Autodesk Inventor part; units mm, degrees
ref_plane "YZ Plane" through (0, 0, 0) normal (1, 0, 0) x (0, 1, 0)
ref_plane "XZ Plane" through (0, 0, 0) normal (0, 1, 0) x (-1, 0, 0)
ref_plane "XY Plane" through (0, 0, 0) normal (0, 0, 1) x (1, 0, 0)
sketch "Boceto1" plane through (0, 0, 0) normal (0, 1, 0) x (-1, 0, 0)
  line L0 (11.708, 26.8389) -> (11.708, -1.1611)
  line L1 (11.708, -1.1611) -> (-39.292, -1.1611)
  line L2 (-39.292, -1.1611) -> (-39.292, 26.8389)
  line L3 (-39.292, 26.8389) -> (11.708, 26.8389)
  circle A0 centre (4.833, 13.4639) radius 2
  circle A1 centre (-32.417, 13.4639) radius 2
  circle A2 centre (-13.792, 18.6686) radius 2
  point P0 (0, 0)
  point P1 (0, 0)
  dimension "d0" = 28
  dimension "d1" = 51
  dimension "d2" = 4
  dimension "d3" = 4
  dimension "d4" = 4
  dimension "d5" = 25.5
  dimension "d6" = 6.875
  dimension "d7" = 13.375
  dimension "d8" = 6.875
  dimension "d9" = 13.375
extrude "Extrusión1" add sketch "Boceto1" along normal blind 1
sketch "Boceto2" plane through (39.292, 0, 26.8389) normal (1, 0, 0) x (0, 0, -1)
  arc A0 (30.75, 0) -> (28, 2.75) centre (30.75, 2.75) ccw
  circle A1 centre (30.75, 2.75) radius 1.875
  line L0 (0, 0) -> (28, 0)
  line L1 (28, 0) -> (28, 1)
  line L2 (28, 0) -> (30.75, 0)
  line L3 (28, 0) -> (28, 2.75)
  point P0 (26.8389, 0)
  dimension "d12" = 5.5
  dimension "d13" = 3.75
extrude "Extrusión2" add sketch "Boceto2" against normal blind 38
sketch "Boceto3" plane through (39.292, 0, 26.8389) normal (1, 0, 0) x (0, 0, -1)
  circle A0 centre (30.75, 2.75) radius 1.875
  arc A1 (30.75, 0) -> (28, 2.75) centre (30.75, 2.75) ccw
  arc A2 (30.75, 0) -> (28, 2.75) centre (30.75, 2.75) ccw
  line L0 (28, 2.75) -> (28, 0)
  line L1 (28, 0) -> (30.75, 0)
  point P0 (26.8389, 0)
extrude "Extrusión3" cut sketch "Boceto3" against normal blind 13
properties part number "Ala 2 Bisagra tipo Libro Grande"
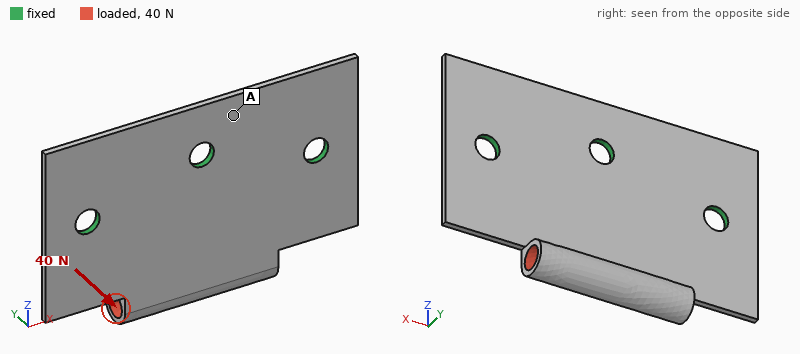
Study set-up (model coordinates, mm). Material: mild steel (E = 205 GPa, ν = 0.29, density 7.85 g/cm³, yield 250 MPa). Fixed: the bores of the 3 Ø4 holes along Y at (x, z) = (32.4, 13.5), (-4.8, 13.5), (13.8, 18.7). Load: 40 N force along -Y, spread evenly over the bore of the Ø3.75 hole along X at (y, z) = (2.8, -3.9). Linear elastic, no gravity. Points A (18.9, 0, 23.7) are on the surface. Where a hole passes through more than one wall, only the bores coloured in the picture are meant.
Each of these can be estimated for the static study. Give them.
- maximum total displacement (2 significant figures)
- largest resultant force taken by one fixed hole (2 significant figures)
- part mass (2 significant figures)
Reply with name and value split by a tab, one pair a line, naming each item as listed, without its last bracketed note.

maximum total displacement	0.12 mm
largest resultant force taken by one fixed hole	22 N
part mass	14 g
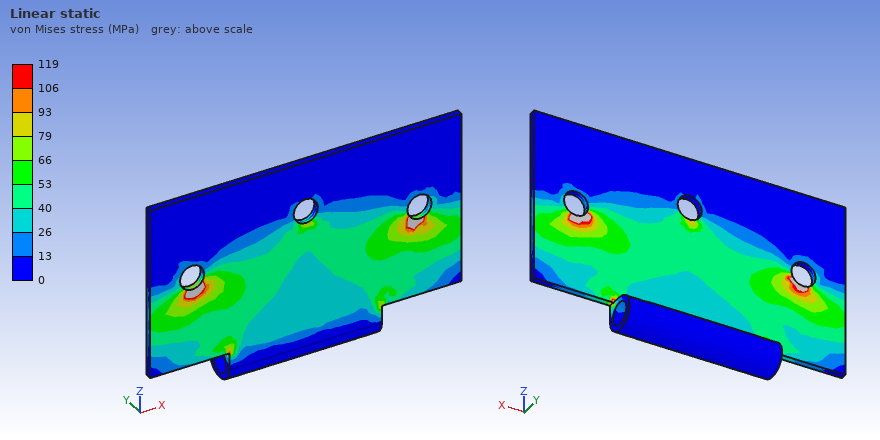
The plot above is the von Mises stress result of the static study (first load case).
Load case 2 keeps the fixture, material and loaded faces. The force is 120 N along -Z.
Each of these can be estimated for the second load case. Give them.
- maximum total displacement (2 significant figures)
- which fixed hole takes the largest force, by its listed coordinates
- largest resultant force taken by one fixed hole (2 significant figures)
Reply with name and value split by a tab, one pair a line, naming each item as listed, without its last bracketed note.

maximum total displacement	70 µm
which fixed hole takes the largest force, by its listed coordinates	(13.8, 18.7)
largest resultant force taken by one fixed hole	64 N
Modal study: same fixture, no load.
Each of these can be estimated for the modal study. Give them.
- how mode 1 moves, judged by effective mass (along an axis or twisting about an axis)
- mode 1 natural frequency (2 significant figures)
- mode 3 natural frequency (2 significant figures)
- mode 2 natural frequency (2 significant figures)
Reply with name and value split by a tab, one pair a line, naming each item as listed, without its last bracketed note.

how mode 1 moves, judged by effective mass	along Y
mode 1 natural frequency	1700 Hz
mode 3 natural frequency	6400 Hz
mode 2 natural frequency	4400 Hz
